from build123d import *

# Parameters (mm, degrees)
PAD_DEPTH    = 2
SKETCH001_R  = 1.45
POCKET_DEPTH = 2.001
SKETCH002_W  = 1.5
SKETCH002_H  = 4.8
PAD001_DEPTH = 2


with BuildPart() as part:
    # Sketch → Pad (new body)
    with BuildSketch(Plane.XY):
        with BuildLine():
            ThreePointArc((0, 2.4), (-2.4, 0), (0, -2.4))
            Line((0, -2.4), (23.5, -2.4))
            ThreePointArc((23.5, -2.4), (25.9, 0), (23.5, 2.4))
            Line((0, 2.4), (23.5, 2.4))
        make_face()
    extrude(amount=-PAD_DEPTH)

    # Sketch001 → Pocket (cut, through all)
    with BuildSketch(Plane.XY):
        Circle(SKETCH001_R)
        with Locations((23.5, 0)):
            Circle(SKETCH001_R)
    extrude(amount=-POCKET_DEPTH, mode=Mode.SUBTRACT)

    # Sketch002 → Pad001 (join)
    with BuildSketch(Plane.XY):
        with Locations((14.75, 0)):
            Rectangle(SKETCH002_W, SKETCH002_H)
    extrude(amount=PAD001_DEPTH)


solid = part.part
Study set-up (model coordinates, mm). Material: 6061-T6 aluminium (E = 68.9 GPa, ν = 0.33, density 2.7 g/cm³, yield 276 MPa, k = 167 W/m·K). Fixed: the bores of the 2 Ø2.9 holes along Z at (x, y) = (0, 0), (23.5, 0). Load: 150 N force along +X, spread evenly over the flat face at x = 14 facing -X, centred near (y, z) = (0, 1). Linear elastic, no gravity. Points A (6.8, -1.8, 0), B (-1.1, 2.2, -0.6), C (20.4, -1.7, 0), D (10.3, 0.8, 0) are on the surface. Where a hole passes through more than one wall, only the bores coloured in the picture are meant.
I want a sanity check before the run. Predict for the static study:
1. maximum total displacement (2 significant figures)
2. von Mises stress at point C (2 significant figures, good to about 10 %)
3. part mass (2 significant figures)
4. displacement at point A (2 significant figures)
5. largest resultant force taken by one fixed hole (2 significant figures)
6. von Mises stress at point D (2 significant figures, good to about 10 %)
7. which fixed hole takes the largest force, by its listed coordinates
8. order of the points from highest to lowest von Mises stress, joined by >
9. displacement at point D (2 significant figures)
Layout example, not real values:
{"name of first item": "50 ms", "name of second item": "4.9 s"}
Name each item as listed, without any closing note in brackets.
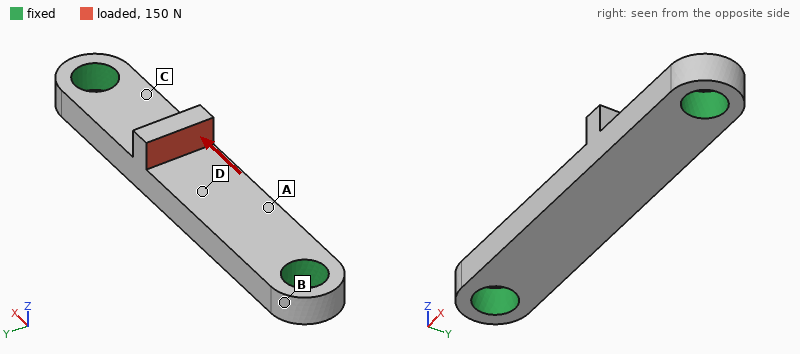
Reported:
{"maximum total displacement": "13 µm", "von Mises stress at point C": "18 MPa", "part mass": "0.67 g", "displacement at point A": "4.8 µm", "largest resultant force taken by one fixed hole": "97 N", "von Mises stress at point D": "31 MPa", "which fixed hole takes the largest force, by its listed coordinates": "(23.5, 0)", "order of the points from highest to lowest von Mises stress, joined by >": "D > C > A > B", "displacement at point D": "7.6 µm"}
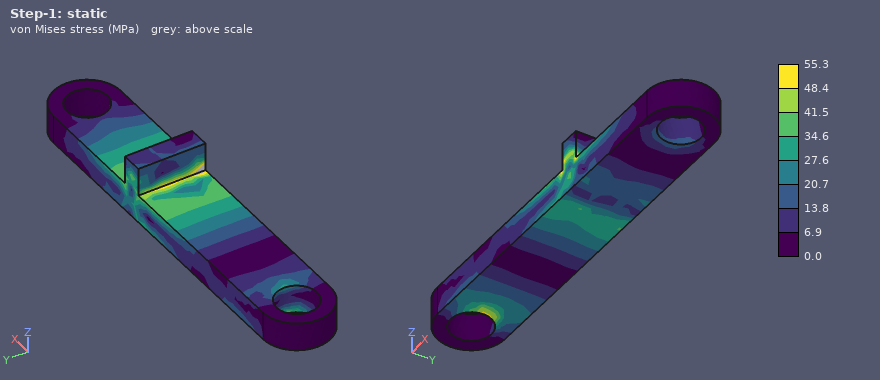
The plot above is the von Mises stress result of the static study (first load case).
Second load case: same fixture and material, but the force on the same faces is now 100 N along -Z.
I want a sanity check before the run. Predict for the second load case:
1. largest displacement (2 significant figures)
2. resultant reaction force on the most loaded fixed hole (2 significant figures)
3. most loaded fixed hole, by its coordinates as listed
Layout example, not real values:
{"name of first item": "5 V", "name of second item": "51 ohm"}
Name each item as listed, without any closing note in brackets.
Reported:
{"largest displacement": "24 µm", "resultant reaction force on the most loaded fixed hole": "65 N", "most loaded fixed hole, by its coordinates as listed": "(23.5, 0)"}
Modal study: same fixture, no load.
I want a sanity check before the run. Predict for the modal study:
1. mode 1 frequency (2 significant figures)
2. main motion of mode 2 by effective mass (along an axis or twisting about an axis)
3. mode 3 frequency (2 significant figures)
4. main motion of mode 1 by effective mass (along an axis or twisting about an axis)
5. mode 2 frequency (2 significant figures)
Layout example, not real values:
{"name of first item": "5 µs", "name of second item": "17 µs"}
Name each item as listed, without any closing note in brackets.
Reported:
{"mode 1 frequency": "21 kHz", "main motion of mode 2 by effective mass": "along Y", "mode 3 frequency": "45 kHz", "main motion of mode 1 by effective mass": "along Z", "mode 2 frequency": "35 kHz"}
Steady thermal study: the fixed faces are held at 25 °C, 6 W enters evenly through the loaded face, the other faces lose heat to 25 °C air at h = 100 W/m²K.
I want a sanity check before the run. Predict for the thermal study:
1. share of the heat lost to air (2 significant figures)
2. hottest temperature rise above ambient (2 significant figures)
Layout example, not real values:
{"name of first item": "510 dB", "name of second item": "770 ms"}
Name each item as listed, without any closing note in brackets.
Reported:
{"share of the heat lost to air": "4.9 %", "hottest temperature rise above ambient": "26 K"}
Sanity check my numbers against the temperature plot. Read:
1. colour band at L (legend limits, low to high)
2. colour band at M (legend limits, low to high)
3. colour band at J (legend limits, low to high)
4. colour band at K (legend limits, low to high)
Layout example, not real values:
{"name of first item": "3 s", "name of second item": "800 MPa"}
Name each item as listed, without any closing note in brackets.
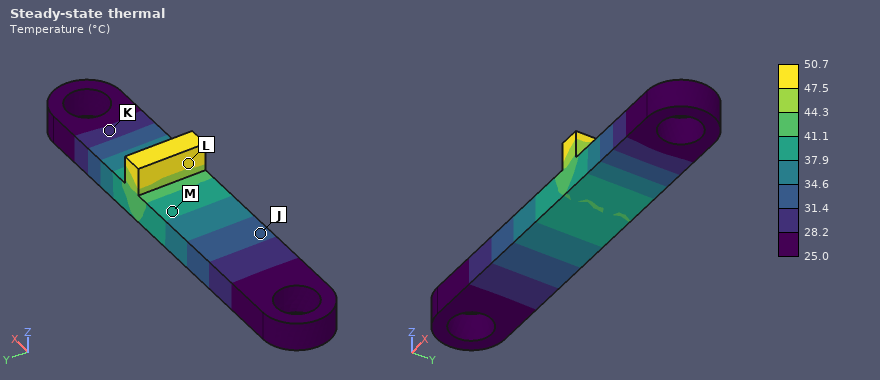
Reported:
{"colour band at L": "47.5 to 50.7 °C", "colour band at M": "37.9 to 41.1 °C", "colour band at J": "31.4 to 34.6 °C", "colour band at K": "28.2 to 31.4 °C"}
